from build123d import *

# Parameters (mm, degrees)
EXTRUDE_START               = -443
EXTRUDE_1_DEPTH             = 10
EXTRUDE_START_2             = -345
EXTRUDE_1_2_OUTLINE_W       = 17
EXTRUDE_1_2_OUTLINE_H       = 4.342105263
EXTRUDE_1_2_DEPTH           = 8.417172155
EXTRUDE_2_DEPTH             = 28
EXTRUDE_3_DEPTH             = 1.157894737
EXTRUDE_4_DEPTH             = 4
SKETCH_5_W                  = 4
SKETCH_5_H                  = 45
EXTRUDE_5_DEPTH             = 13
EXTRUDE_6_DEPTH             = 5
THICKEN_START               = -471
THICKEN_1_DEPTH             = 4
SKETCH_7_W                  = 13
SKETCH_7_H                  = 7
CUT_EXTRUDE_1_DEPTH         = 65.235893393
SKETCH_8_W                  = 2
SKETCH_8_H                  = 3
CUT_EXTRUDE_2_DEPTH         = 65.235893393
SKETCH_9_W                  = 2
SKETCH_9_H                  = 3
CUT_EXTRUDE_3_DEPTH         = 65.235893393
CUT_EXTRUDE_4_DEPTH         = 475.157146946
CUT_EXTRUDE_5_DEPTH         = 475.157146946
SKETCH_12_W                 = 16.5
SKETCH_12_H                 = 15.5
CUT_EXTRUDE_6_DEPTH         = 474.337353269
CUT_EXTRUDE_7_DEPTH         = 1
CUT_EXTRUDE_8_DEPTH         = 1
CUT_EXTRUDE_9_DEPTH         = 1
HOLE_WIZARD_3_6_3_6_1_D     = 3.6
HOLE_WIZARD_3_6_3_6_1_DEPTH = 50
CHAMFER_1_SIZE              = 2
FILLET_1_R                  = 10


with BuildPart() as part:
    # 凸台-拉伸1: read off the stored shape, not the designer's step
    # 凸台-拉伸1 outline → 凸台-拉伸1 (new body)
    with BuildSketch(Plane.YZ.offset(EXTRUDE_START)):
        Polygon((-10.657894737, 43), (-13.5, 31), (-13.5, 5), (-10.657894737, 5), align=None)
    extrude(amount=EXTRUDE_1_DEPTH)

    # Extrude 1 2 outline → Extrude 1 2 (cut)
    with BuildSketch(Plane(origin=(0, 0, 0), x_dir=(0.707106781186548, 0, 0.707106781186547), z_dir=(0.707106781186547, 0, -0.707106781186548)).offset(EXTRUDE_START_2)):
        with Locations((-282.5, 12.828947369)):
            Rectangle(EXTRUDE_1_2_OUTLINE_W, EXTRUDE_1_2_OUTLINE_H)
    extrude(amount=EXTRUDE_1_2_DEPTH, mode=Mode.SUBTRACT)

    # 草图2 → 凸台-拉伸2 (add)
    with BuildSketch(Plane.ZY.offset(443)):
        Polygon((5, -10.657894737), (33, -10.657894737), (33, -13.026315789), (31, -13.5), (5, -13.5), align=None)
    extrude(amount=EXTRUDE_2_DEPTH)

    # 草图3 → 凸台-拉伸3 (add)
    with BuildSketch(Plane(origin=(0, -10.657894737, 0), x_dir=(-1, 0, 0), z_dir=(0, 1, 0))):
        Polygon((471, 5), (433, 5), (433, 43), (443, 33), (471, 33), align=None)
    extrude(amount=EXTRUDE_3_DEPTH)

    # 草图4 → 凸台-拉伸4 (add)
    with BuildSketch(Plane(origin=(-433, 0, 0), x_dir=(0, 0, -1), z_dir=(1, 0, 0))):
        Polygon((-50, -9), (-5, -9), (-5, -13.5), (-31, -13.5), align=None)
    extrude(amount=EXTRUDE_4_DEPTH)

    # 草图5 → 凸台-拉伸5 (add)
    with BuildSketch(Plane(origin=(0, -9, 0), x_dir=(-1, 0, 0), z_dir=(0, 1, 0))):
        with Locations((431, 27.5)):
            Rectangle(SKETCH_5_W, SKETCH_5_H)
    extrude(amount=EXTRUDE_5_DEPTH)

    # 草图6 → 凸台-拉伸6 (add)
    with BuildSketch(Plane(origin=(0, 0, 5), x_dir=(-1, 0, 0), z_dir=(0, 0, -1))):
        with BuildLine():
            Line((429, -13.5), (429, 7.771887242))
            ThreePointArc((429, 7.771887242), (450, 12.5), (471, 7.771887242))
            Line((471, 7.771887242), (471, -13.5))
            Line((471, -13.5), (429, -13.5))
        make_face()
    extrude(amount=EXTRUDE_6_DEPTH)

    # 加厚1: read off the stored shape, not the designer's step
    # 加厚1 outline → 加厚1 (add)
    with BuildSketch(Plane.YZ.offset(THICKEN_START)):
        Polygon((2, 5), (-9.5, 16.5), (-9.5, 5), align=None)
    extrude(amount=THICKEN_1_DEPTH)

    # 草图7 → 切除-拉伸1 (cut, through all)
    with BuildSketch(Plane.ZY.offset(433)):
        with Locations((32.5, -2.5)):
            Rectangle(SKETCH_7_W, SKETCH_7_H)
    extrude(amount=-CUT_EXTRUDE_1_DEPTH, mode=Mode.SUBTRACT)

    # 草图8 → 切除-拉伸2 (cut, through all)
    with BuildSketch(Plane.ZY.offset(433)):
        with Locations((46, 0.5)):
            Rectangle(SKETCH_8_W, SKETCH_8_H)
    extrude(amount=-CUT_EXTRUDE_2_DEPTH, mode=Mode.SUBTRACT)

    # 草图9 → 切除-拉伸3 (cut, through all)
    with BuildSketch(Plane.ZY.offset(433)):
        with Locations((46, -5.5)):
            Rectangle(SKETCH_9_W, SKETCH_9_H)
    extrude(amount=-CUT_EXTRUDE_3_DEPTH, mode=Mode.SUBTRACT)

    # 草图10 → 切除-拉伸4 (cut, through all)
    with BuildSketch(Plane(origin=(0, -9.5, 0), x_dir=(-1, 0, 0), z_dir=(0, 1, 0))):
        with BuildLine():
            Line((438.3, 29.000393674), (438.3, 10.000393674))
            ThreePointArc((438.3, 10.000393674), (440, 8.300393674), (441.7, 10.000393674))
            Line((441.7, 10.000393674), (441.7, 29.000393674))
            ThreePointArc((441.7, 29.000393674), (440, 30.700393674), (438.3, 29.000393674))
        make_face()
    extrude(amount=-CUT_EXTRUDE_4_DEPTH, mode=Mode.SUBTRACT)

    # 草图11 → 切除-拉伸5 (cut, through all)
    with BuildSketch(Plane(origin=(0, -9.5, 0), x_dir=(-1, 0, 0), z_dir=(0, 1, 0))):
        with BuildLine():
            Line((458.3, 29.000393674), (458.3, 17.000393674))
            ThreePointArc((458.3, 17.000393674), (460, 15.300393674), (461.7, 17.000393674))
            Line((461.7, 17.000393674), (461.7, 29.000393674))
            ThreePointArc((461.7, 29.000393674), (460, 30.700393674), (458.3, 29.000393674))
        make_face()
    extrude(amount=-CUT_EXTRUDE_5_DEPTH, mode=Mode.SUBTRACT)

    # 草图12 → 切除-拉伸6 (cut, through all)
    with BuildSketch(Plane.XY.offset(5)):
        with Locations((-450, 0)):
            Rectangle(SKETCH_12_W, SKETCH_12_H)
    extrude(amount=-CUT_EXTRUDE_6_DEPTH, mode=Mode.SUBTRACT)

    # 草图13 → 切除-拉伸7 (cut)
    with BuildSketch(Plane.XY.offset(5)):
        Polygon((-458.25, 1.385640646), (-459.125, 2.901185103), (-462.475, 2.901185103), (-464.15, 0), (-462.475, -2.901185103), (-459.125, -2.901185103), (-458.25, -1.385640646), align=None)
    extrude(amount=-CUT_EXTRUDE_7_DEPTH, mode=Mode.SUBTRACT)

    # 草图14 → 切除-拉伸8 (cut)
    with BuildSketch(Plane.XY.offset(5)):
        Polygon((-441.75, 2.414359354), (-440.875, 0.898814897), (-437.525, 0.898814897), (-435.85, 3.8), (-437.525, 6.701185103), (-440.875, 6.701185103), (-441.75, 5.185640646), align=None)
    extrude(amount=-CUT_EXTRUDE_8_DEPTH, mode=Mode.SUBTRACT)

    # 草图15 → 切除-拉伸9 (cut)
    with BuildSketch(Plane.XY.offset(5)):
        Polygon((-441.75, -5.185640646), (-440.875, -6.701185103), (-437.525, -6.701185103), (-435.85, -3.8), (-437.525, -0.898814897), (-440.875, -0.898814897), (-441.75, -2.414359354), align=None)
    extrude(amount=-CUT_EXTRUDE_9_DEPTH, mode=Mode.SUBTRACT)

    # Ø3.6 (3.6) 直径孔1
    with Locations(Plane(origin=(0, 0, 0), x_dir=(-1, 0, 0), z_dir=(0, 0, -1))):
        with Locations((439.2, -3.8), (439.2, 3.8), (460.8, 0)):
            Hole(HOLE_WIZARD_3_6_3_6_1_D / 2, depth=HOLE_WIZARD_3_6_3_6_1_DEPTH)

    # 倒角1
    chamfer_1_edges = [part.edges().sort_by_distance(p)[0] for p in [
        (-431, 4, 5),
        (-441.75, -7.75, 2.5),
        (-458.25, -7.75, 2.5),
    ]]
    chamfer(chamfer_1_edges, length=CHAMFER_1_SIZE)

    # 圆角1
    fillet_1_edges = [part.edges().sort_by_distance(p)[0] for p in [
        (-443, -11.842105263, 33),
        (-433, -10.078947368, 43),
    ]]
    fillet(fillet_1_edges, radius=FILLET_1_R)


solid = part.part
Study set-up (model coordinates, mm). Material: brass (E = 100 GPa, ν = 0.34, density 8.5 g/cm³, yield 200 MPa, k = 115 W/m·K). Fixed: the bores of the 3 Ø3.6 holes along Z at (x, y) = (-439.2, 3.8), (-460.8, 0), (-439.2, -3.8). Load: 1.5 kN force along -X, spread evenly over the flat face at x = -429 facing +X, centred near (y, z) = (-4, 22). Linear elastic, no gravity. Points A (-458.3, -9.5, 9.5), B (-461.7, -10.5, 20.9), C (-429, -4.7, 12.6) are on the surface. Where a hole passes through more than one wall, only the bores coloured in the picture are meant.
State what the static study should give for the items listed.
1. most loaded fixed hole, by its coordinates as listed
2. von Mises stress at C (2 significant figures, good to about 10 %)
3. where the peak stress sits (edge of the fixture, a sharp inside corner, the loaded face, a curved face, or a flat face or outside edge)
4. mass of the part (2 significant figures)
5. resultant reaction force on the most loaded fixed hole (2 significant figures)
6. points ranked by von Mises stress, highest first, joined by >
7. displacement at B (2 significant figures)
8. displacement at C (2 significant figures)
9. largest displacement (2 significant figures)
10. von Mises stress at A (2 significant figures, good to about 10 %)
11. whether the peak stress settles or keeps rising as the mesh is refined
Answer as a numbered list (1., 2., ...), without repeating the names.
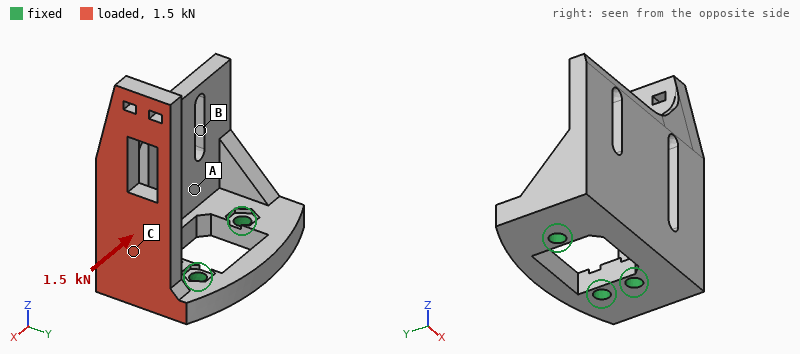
1. (-439.2, -3.8)
2. 69 MPa
3. edge of the fixture
4. 88 g
5. 1.3 kN
6. C > A > B
7. 0.074 mm
8. 0.047 mm
9. 0.31 mm
10. 44 MPa
11. keeps rising
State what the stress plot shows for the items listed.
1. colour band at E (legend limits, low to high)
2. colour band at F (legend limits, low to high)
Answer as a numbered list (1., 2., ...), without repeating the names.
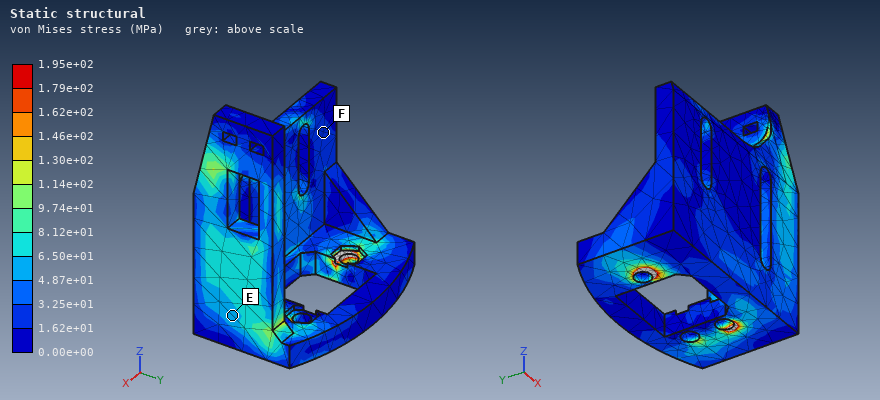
1. 4.87e+01 to 6.50e+01 MPa
2. 1.62e+01 to 3.25e+01 MPa
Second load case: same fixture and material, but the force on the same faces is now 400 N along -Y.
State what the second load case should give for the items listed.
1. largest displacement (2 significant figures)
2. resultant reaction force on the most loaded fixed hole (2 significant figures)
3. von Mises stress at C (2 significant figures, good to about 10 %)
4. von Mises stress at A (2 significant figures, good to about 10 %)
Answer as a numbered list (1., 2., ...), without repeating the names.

1. 81 µm
2. 670 N
3. 15 MPa
4. 10 MPa
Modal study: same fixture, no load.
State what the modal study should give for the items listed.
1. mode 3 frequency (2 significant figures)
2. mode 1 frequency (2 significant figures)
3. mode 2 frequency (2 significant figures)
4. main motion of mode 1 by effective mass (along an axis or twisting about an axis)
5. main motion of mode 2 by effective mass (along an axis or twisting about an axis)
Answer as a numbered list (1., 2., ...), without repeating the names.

1. 4700 Hz
2. 2200 Hz
3. 2400 Hz
4. along Y
5. along X
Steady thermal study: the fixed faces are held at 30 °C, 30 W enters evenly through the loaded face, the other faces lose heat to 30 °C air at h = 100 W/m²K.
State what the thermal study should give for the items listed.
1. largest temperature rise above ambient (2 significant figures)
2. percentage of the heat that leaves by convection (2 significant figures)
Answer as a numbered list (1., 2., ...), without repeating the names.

1. 48 K
2. 27 %
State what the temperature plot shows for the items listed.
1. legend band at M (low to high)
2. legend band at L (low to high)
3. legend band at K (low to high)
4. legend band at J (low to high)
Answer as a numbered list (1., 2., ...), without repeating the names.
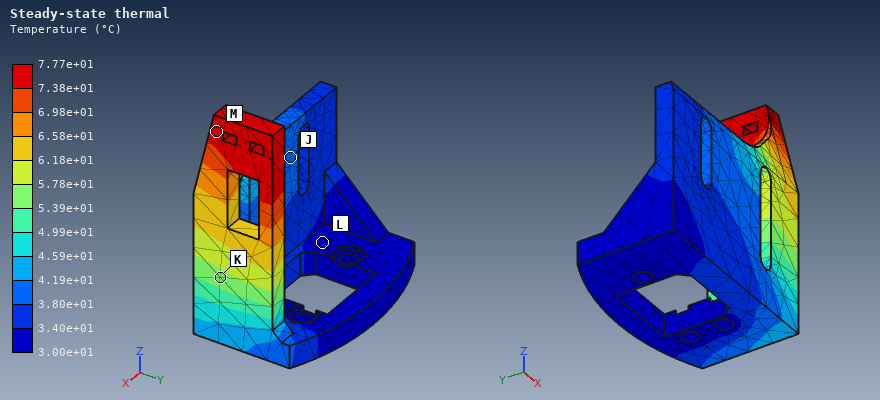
1. 7.38e+01 to 7.77e+01 °C
2. 3.00e+01 to 3.40e+01 °C
3. 5.39e+01 to 5.78e+01 °C
4. 3.80e+01 to 4.19e+01 °C
